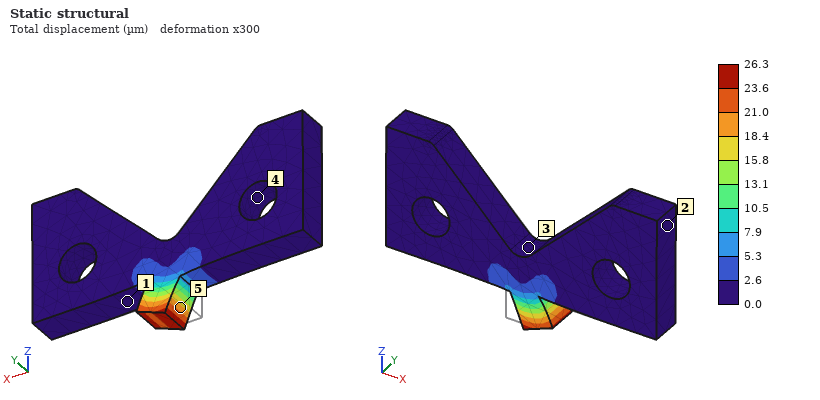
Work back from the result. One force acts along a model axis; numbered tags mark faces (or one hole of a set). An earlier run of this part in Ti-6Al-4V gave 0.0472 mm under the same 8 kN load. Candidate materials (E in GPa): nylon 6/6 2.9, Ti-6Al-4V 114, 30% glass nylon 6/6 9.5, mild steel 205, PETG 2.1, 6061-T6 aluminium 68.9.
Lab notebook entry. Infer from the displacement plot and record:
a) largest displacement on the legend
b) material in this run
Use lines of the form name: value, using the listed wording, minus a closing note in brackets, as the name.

largest displacement on the legend: 26.3 µm
material in this run: mild steel
